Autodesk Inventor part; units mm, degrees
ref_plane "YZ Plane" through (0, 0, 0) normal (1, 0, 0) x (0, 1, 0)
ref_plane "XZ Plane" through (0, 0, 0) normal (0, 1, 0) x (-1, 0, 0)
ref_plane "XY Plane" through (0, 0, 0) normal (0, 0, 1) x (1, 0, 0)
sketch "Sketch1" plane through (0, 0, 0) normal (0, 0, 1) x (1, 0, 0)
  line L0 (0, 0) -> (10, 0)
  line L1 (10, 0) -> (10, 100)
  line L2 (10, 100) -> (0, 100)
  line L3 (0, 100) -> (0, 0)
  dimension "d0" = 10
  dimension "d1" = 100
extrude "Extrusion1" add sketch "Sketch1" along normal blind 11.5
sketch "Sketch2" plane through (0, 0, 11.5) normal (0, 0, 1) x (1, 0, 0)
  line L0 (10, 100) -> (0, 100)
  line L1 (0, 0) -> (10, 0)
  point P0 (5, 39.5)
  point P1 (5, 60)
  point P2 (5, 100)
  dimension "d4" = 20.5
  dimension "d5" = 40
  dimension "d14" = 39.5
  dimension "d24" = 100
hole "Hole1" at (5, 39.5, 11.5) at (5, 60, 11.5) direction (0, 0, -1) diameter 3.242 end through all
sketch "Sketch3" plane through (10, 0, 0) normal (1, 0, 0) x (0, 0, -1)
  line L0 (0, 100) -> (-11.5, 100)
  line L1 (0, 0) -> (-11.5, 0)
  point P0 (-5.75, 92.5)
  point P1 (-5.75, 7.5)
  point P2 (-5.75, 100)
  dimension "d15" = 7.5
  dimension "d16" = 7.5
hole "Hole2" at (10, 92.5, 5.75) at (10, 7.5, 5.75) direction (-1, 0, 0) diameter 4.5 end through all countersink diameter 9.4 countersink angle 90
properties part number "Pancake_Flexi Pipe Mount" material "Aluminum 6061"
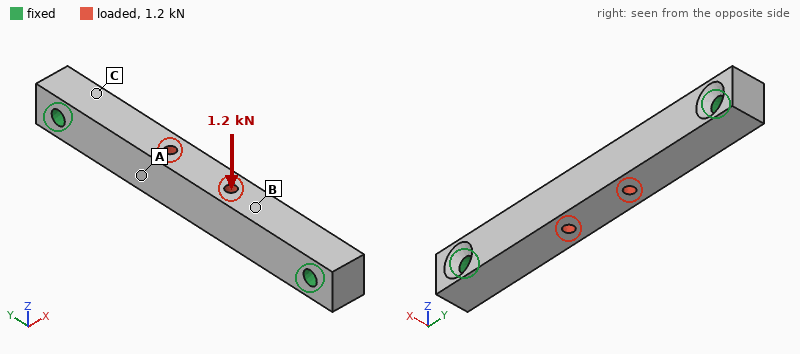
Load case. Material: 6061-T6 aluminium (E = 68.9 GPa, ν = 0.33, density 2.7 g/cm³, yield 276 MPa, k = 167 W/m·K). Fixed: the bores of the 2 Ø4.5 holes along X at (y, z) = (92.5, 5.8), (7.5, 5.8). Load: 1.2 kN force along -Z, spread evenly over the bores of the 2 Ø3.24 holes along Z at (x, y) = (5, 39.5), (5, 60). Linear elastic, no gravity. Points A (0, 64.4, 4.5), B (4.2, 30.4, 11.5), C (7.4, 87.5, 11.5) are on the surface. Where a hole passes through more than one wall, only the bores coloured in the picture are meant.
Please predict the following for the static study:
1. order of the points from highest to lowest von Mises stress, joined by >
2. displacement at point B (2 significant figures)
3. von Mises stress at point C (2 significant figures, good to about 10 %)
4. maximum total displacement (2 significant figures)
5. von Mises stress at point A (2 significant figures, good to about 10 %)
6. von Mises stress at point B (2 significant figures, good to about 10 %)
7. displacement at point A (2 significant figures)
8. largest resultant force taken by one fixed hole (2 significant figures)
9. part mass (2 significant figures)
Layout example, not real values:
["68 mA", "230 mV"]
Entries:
["C > A > B", "39 µm", "36 MPa", "59 µm", "18 MPa", "11 MPa", "47 µm", "600 N", "29 g"]
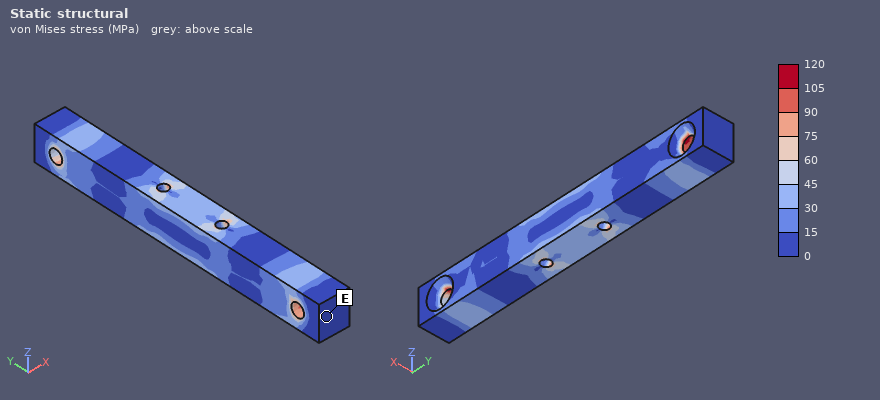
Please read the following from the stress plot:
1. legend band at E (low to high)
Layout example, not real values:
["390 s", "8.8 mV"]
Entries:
["0 to 15 MPa"]
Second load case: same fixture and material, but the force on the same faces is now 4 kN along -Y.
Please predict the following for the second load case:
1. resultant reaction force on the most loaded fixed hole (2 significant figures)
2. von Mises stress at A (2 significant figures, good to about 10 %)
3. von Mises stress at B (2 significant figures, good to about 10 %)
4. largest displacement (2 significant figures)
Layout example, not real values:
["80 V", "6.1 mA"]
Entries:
["2.0 kN", "17 MPa", "18 MPa", "9.5 µm"]
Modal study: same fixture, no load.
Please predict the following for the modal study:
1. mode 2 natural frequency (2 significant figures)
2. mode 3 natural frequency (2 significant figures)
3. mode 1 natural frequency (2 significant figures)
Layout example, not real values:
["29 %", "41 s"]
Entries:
["6500 Hz", "16 kHz", "6400 Hz"]
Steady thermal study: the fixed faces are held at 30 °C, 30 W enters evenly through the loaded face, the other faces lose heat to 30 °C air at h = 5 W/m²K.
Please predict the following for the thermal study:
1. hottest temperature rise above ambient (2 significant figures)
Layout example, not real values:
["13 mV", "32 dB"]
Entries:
["26 K"]
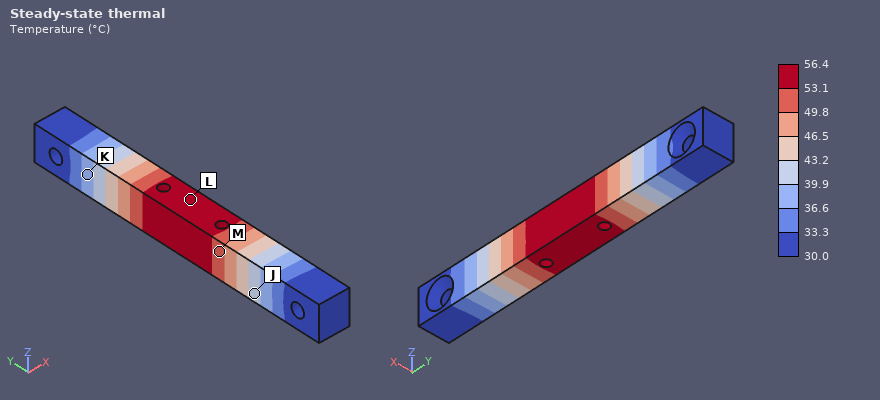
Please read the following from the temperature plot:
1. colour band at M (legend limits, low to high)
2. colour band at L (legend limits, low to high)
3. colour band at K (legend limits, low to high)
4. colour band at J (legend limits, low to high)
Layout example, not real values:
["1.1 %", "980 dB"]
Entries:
["49.8 to 53.1 °C", "53.1 to 56.4 °C", "36.6 to 39.9 °C", "39.9 to 43.2 °C"]
